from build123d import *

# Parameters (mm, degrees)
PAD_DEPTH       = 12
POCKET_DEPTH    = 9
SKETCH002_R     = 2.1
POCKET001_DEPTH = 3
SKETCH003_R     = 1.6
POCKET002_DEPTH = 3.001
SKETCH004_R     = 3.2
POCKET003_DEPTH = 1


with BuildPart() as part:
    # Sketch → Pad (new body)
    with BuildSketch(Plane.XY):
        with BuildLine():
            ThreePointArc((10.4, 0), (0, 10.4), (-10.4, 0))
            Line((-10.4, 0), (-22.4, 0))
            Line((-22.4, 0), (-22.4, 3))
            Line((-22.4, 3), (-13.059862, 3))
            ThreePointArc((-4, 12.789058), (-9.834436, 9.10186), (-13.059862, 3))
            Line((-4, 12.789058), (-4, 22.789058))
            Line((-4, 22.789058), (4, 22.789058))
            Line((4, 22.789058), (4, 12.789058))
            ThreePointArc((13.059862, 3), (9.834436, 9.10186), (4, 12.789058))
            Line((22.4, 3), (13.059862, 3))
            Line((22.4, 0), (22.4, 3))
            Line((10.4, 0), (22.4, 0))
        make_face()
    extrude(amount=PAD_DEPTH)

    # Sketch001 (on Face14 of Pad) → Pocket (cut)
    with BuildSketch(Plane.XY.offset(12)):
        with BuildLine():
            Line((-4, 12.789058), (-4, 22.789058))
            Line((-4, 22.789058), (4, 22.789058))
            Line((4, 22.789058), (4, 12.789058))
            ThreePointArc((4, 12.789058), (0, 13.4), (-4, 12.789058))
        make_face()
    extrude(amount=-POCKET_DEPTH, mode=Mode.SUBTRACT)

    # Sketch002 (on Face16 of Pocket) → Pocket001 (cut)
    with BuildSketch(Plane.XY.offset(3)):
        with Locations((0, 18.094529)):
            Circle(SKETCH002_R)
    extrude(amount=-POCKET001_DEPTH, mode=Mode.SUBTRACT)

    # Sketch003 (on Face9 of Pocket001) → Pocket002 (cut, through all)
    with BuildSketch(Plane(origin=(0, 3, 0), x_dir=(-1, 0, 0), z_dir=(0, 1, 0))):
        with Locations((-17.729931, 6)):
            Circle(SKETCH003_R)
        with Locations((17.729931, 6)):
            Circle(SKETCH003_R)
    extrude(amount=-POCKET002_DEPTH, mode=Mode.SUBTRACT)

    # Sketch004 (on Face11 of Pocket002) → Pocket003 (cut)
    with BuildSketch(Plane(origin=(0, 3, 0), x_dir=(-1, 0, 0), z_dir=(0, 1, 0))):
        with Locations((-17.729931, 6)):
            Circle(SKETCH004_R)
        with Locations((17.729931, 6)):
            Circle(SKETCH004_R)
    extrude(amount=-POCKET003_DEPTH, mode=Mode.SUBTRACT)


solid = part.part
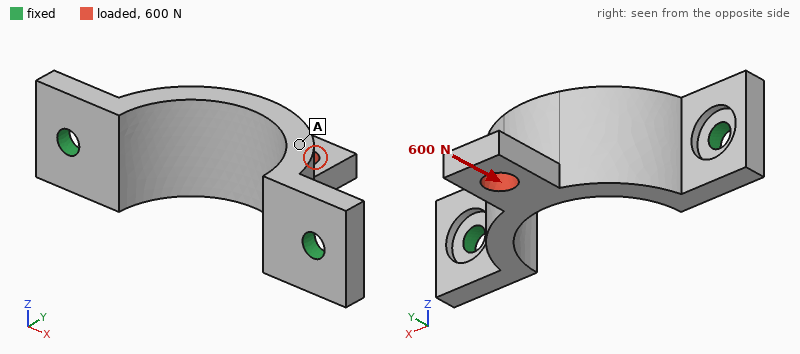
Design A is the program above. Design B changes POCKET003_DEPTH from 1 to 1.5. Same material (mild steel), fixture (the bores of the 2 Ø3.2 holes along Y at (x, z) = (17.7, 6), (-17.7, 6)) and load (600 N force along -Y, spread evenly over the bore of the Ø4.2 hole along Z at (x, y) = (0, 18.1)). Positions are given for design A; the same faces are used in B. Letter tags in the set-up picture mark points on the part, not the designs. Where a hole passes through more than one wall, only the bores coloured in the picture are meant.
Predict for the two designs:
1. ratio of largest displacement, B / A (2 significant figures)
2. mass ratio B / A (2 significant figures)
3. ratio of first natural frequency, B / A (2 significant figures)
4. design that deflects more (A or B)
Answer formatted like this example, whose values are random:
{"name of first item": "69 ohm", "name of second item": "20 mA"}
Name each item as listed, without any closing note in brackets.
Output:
{"ratio of largest displacement, B / A": "1.3", "mass ratio B / A": "0.99", "ratio of first natural frequency, B / A": "0.85", "design that deflects more": "B"}
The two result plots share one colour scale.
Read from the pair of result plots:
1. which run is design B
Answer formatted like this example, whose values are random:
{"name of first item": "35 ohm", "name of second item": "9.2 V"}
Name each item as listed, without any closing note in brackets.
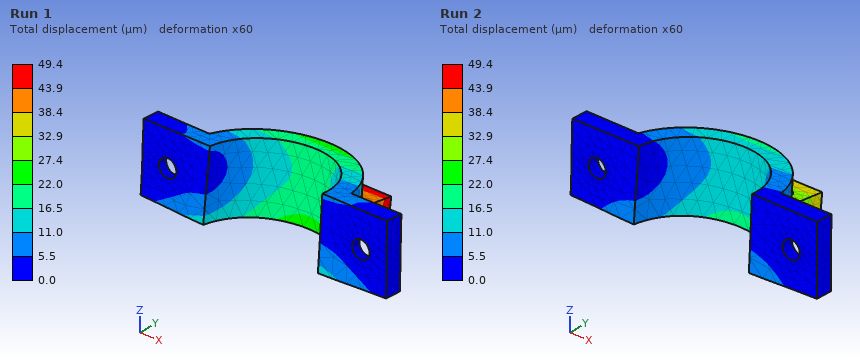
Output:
{"which run is design B": "Run 1"}
